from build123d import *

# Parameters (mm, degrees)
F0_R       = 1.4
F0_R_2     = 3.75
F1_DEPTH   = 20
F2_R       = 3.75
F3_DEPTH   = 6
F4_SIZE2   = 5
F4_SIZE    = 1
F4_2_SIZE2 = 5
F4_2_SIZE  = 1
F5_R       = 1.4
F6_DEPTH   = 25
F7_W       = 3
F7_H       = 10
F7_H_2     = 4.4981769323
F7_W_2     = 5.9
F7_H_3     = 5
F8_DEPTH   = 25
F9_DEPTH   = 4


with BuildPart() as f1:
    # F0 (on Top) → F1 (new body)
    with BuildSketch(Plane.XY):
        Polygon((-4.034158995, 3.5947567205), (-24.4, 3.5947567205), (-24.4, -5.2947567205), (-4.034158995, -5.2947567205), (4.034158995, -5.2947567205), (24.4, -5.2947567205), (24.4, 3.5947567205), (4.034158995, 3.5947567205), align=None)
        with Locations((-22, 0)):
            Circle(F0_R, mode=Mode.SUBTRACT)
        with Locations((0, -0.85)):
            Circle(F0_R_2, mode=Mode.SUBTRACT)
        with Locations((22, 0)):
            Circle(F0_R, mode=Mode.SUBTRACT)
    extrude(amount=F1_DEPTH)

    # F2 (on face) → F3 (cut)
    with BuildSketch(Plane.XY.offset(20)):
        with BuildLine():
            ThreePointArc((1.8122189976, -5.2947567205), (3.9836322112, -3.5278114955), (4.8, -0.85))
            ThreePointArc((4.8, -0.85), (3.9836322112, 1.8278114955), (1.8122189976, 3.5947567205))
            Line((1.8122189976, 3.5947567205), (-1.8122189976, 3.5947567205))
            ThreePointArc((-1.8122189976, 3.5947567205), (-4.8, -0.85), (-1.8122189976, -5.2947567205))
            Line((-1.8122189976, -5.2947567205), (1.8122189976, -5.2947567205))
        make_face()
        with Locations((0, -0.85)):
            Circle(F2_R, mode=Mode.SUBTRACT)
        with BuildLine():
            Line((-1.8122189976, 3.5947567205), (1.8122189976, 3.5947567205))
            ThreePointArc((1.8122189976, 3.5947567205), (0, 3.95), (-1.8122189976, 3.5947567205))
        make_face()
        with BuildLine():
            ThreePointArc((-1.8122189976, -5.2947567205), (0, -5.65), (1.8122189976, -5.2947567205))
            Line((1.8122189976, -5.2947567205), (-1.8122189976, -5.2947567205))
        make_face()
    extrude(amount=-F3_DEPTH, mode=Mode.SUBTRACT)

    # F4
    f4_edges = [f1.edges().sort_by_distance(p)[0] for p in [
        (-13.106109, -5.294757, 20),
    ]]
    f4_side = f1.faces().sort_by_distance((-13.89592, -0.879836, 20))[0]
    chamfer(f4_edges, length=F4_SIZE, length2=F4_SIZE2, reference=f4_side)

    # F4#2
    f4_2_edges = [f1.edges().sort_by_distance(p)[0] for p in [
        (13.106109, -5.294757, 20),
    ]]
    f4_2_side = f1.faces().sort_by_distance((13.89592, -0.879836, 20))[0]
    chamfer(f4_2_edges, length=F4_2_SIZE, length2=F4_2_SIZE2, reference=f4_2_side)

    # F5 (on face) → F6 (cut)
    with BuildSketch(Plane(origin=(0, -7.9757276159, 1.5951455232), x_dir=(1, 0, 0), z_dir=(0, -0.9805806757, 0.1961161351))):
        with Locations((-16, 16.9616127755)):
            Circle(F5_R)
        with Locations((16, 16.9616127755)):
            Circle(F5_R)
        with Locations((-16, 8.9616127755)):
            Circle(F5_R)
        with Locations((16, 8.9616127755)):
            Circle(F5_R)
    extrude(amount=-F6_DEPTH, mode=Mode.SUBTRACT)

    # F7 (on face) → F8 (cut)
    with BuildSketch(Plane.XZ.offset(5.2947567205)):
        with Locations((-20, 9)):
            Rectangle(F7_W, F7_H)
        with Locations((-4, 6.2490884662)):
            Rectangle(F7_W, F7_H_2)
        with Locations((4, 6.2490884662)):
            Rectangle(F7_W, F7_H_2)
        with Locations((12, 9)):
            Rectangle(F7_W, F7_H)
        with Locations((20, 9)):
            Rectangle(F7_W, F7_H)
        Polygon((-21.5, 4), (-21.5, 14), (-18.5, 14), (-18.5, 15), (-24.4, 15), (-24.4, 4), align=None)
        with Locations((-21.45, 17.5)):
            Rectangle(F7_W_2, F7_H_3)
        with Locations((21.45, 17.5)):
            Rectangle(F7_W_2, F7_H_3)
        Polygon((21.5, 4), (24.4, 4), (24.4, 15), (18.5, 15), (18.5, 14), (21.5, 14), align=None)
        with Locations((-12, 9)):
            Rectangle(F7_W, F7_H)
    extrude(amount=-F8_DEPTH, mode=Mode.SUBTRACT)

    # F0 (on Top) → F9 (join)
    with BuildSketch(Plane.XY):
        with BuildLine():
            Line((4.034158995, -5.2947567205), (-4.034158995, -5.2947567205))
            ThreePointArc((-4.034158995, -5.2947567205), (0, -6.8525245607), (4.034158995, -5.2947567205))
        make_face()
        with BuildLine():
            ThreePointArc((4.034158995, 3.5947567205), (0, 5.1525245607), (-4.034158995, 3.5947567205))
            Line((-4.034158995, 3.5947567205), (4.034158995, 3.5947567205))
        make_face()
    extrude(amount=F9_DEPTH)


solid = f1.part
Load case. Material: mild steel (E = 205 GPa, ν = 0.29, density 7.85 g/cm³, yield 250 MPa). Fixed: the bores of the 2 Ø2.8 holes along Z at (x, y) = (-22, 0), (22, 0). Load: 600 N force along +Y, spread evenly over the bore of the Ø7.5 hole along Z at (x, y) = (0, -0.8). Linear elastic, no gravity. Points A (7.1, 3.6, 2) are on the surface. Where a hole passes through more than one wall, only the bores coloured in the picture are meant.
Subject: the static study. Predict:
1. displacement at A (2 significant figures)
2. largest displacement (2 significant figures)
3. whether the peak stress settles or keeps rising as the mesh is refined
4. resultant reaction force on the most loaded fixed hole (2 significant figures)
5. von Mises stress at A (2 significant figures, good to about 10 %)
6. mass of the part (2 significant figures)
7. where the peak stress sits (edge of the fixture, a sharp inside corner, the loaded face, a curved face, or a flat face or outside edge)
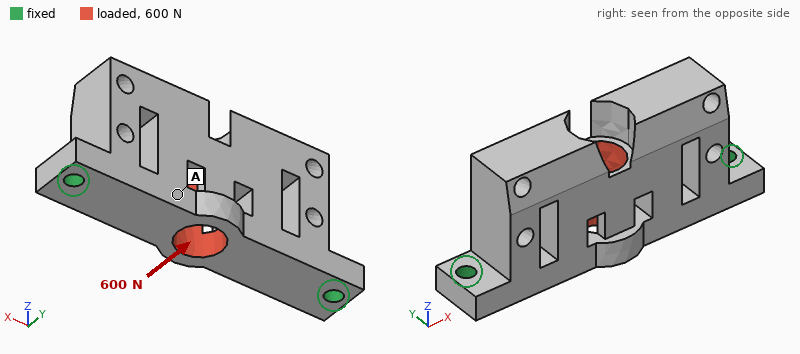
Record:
6.0 µm
19 µm
keeps rising
300 N
23 MPa
39 g
edge of the fixture
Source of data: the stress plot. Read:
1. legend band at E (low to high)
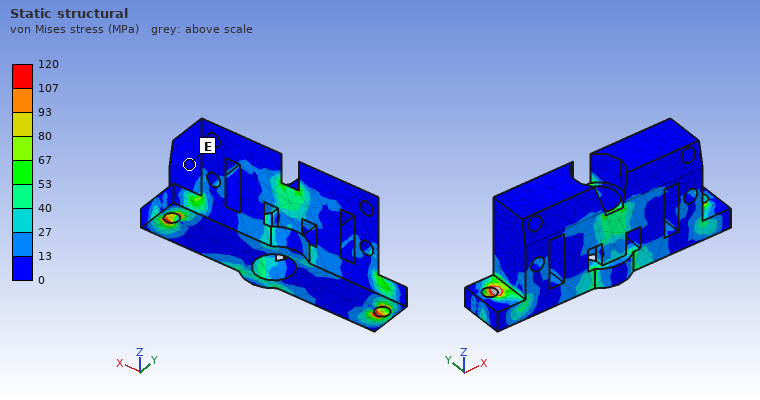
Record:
0 to 13 MPa
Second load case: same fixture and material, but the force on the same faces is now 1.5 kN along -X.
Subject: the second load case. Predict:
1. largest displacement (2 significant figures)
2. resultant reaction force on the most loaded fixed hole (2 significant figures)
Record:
3.7 µm
770 N
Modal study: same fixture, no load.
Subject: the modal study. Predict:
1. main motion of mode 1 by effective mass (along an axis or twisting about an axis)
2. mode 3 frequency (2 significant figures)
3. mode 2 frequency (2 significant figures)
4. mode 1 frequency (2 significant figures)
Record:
along Y
11 kHz
11 kHz
5300 Hz
